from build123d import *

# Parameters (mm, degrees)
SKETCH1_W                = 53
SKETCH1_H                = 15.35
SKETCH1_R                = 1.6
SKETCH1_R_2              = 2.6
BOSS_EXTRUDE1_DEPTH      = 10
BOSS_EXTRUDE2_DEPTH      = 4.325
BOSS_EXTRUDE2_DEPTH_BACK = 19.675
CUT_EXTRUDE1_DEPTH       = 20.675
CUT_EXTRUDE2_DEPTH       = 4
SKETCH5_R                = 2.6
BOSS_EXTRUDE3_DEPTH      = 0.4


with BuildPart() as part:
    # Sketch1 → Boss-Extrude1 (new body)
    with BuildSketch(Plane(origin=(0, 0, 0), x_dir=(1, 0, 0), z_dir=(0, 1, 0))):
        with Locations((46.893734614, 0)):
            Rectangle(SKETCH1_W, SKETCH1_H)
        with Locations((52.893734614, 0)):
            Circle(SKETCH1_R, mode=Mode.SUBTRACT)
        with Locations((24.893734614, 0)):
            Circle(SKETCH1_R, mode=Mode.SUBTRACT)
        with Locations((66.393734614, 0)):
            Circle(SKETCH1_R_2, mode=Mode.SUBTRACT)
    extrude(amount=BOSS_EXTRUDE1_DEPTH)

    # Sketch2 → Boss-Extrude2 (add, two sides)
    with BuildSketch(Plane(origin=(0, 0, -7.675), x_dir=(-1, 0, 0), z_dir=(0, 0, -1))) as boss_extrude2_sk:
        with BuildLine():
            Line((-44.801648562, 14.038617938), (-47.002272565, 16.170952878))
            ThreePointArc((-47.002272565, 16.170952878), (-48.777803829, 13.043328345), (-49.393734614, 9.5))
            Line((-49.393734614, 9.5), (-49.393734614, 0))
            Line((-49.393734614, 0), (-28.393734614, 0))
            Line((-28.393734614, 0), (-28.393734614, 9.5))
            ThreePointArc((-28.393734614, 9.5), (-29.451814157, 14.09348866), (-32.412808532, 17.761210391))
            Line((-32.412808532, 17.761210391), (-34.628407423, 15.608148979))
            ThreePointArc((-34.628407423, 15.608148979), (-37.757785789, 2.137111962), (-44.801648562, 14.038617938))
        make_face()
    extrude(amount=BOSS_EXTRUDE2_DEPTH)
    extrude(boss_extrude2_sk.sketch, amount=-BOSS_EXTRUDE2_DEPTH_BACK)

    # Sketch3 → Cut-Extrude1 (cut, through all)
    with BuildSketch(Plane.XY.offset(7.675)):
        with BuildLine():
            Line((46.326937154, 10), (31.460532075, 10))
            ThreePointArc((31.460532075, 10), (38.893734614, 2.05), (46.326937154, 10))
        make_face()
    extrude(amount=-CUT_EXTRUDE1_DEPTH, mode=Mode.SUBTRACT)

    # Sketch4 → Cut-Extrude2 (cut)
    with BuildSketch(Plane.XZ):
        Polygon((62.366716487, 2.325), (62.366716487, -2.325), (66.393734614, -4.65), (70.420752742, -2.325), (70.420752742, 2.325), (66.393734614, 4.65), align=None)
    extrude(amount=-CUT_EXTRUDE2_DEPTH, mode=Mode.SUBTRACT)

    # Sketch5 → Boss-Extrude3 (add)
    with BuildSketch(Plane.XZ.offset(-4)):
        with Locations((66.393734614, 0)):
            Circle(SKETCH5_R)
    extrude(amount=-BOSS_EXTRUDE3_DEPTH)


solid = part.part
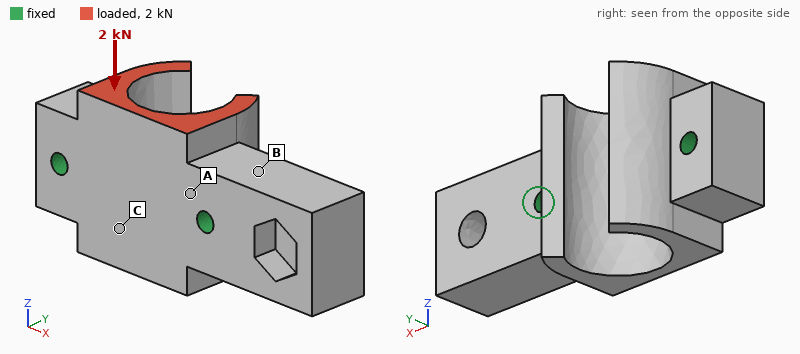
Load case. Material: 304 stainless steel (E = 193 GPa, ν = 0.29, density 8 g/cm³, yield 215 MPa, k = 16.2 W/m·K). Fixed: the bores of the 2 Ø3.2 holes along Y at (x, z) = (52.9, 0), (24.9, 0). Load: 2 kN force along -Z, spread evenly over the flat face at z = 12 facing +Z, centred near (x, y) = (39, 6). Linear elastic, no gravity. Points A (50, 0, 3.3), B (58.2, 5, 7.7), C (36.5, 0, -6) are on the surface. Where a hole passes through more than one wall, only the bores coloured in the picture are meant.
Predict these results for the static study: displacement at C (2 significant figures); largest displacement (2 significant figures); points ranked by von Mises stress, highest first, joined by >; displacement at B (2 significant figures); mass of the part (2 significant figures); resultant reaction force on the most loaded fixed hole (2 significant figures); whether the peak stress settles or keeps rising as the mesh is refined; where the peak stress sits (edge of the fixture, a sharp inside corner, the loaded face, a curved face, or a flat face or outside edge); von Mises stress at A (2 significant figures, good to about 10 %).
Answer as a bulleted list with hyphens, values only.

- 1.2 µm
- 4.1 µm
- A > C > B
- 0.69 µm
- 65 g
- 1.0 kN
- keeps rising
- edge of the fixture
- 17 MPa
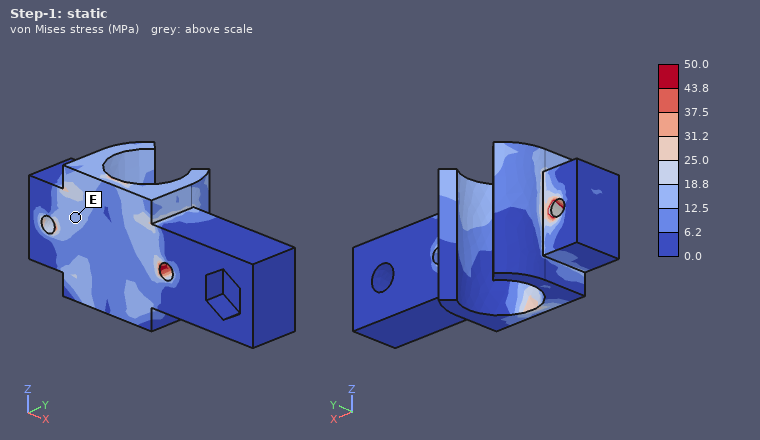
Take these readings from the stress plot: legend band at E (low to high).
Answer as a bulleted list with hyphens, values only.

- 12.5 to 18.8 MPa
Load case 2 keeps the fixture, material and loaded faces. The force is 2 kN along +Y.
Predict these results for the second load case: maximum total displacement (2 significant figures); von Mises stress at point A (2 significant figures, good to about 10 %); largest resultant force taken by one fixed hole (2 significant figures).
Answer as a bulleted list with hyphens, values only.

- 15 µm
- 62 MPa
- 1.1 kN
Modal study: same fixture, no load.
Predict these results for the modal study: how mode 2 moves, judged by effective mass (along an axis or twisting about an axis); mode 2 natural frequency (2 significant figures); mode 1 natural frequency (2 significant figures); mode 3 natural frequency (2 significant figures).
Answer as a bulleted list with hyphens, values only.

- along Y
- 15 kHz
- 15 kHz
- 22 kHz
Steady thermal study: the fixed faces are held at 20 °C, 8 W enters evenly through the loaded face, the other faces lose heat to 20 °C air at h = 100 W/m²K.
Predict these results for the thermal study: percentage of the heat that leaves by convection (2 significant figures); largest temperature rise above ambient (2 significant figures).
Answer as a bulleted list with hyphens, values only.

- 32 %
- 32 K
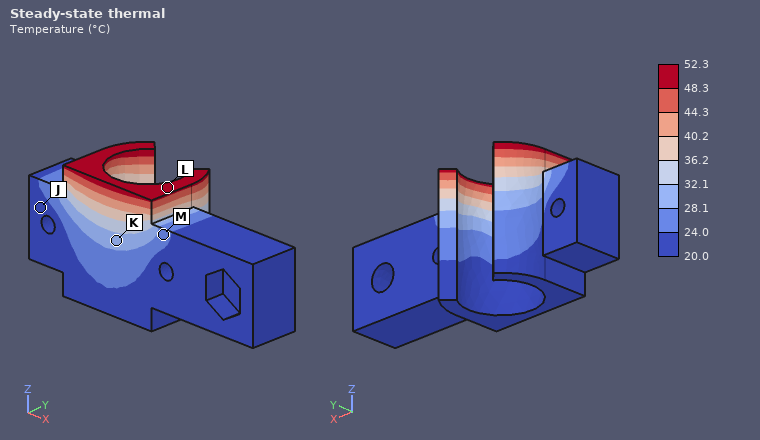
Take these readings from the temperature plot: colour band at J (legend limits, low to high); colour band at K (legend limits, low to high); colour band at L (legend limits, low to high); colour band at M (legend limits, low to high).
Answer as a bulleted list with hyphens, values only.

- 20.0 to 24.0 °C
- 28.1 to 32.1 °C
- 48.3 to 52.3 °C
- 24.0 to 28.1 °C
